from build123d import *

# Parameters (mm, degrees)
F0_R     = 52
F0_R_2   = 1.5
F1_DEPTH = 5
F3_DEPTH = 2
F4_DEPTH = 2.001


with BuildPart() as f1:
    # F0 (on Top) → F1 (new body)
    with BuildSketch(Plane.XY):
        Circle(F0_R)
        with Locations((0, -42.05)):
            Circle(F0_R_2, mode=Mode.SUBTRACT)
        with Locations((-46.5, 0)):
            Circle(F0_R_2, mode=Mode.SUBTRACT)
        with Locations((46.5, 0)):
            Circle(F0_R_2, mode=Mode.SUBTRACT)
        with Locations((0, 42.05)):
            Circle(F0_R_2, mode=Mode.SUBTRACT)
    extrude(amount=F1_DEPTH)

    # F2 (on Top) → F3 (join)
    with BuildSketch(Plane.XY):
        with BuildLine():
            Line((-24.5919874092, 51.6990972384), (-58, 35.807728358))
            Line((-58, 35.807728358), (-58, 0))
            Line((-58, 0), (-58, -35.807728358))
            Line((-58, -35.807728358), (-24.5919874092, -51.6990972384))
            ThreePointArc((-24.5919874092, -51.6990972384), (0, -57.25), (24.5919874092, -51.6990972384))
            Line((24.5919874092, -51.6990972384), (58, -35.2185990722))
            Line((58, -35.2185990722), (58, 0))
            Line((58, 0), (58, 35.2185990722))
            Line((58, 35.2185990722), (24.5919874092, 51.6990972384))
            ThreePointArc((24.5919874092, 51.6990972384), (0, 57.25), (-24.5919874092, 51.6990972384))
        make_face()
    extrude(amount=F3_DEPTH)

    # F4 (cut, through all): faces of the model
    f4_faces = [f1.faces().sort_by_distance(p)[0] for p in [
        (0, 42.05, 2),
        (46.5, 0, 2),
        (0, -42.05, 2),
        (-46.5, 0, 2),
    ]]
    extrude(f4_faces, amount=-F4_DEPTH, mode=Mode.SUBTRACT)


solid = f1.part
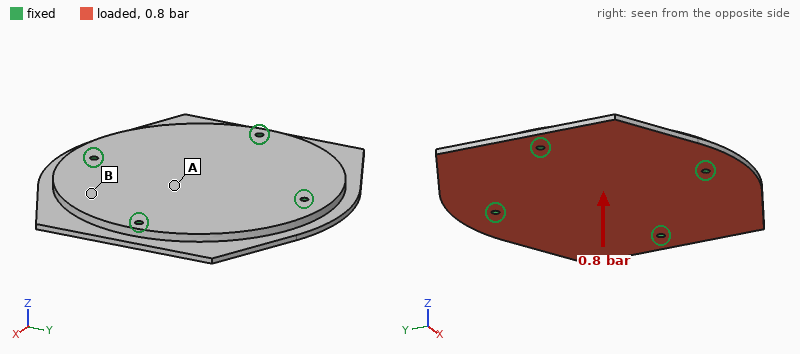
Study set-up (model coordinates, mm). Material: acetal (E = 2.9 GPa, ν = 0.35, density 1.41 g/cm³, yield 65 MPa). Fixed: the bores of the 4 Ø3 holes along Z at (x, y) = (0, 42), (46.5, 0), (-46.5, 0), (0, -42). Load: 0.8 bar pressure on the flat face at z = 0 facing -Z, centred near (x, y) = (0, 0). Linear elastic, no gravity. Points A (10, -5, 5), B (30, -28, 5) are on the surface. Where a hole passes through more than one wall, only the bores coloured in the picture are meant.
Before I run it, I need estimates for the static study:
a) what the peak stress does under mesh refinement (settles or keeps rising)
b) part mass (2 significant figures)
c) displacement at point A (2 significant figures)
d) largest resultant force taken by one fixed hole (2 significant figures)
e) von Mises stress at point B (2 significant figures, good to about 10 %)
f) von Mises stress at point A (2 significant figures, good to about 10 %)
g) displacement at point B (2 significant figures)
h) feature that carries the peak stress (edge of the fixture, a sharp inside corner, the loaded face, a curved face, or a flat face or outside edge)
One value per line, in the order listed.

keeps rising
68 g
0.22 mm
230 N
5.6 MPa
2.2 MPa
0.25 mm
edge of the fixture
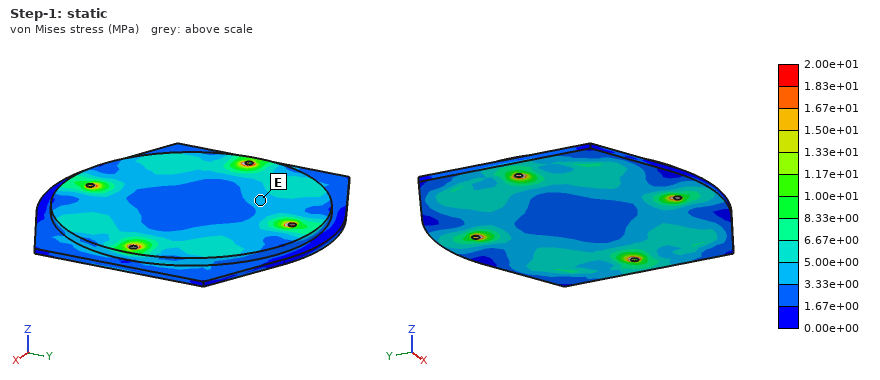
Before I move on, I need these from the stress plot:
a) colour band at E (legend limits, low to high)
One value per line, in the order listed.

3.33e+00 to 5.00e+00 MPa
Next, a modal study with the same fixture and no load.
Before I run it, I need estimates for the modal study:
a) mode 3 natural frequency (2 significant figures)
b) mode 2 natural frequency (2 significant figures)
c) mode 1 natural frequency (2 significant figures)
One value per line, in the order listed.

1100 Hz
1100 Hz
1000 Hz
